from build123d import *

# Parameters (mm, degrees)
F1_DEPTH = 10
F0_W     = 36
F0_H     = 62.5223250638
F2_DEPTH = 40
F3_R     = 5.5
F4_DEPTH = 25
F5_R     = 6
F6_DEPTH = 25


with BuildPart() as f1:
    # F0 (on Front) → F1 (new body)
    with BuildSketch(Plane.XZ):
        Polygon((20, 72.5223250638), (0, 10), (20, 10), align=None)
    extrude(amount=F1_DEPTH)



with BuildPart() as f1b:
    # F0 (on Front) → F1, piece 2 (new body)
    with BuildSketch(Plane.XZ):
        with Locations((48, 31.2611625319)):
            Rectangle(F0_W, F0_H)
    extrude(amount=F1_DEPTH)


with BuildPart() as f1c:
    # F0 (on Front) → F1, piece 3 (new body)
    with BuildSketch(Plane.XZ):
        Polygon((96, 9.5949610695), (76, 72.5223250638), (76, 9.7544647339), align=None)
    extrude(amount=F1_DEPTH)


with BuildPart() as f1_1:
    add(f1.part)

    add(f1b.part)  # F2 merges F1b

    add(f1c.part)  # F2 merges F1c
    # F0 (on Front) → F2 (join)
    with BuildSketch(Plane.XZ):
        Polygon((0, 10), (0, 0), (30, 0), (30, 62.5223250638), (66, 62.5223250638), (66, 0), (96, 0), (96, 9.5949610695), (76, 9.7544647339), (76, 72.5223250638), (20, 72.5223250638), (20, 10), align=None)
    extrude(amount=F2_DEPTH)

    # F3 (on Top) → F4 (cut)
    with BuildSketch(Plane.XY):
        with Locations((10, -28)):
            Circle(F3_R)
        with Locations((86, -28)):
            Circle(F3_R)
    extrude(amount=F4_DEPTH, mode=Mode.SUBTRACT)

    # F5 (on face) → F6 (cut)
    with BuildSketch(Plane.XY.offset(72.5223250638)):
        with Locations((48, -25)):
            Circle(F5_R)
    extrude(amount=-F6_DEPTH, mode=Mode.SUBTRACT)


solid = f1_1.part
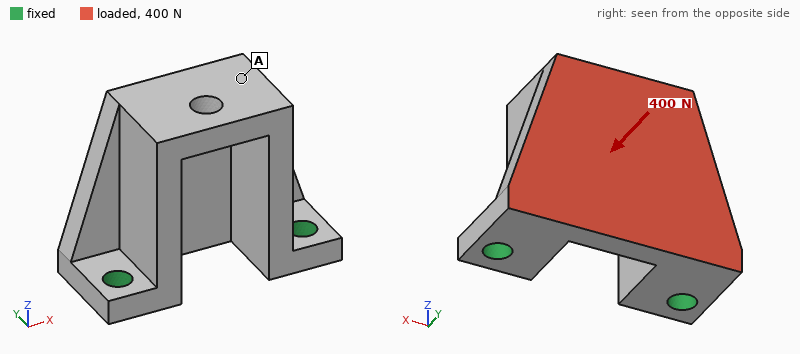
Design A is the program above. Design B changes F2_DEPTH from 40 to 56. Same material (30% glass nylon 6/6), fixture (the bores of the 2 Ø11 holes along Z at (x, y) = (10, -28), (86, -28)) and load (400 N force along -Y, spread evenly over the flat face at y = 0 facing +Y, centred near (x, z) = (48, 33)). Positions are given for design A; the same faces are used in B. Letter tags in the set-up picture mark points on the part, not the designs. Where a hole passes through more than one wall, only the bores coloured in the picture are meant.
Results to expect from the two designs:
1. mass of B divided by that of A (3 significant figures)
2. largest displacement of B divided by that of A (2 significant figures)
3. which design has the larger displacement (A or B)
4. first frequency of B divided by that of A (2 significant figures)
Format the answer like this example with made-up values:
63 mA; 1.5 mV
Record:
1.29; 0.77; A; 0.98
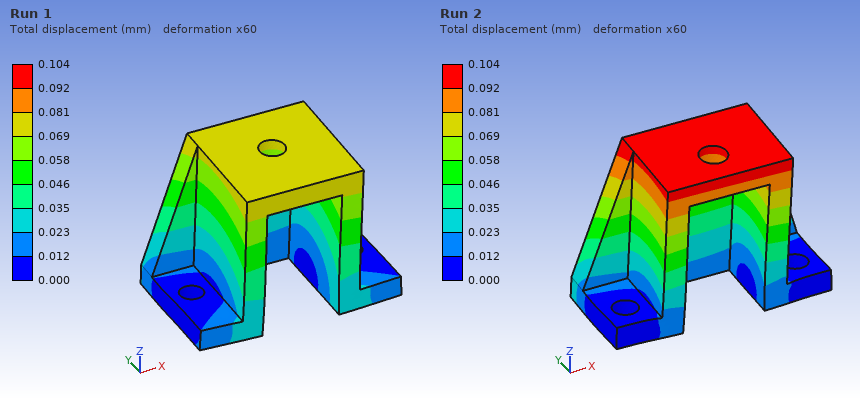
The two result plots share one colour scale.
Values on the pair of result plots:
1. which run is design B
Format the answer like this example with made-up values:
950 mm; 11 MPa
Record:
Run 1
